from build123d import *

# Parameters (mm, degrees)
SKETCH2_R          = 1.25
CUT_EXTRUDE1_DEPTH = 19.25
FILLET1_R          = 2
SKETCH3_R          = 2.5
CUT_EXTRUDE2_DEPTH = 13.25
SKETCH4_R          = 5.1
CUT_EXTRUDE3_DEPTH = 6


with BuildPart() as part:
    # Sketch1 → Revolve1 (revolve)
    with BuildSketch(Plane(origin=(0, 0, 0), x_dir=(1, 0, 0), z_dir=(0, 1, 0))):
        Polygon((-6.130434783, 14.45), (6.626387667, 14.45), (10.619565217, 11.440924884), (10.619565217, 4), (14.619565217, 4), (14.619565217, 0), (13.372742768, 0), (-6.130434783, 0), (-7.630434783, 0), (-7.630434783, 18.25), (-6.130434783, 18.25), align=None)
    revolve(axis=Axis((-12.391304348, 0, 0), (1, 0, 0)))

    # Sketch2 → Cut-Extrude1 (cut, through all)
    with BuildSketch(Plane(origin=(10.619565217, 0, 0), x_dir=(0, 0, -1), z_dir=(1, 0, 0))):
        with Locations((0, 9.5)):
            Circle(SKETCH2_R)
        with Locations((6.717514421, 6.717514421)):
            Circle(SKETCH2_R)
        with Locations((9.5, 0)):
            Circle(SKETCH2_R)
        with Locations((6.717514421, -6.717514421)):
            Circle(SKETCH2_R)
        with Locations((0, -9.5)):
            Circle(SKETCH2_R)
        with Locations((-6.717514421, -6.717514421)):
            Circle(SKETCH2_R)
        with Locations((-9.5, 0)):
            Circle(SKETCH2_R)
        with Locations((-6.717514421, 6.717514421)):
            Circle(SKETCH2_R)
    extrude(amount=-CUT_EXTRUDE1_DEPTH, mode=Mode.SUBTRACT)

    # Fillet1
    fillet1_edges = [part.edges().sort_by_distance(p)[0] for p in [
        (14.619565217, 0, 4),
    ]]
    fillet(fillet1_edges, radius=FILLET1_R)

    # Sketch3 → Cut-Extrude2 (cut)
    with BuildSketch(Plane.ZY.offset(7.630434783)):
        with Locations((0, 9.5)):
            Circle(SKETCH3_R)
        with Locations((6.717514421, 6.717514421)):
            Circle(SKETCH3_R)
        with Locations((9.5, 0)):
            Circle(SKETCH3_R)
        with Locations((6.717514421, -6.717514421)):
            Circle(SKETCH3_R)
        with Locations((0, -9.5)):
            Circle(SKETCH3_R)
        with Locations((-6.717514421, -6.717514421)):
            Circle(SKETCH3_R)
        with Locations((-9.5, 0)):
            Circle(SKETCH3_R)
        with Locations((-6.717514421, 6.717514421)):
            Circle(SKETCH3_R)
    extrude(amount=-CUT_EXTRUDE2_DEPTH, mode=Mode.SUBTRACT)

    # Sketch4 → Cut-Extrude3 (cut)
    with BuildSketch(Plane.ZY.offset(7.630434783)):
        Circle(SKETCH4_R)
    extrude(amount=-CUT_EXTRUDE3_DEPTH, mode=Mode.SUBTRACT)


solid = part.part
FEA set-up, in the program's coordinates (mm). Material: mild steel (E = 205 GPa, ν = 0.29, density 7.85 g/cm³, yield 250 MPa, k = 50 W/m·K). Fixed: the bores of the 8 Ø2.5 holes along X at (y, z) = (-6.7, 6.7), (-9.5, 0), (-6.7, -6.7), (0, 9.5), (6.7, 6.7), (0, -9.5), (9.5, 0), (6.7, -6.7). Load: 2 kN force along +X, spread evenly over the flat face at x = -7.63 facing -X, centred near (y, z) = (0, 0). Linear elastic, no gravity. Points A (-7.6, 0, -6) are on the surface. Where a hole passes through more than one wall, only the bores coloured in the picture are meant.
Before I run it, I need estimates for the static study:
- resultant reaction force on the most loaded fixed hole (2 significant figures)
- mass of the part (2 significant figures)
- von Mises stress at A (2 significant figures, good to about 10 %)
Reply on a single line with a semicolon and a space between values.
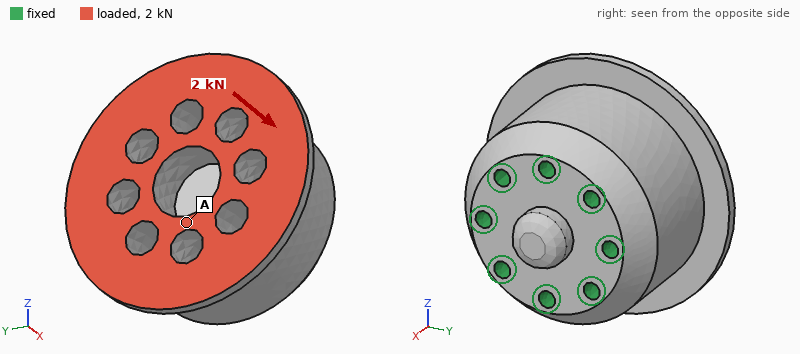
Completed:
250 N; 74 g; 8.5 MPa
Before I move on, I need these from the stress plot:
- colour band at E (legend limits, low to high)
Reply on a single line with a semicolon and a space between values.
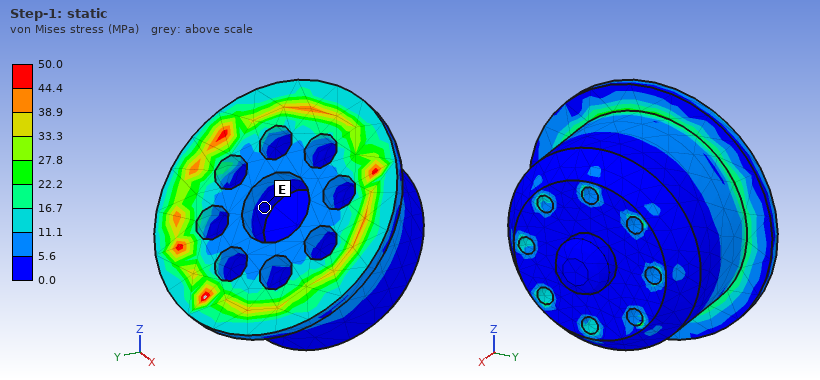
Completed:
0.0 to 5.6 MPa
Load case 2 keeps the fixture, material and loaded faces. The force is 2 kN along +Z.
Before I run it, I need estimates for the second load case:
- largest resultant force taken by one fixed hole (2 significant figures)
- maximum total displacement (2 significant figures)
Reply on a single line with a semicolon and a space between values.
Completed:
720 N; 4.8 µm
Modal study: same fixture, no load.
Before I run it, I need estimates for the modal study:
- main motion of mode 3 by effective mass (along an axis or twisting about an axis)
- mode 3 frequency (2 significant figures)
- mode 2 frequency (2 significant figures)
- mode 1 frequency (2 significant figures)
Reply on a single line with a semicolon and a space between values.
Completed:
twisting about X; 38 kHz; 28 kHz; 28 kHz
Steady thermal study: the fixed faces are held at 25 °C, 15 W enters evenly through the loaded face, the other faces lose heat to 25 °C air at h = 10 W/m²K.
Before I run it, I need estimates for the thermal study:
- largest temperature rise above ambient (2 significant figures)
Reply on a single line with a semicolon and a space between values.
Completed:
14 K
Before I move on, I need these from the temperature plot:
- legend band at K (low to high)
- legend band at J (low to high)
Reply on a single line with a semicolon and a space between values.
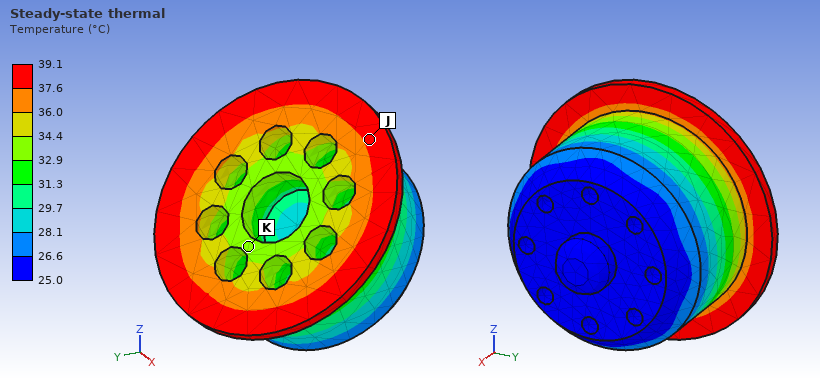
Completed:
32.9 to 34.4 °C; 37.6 to 39.1 °C
